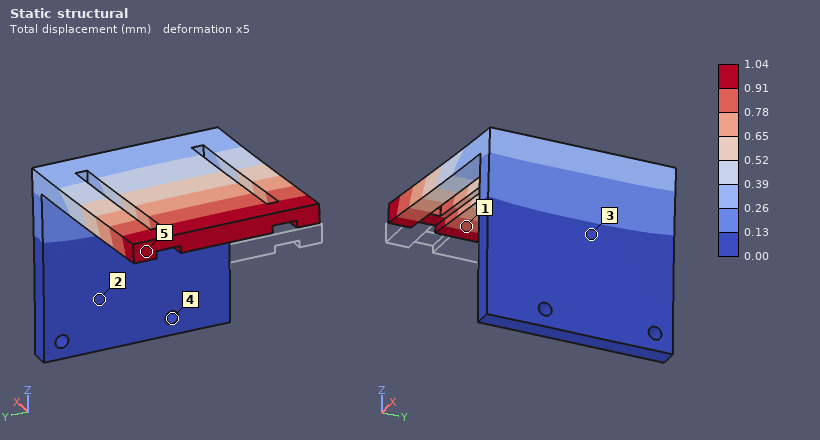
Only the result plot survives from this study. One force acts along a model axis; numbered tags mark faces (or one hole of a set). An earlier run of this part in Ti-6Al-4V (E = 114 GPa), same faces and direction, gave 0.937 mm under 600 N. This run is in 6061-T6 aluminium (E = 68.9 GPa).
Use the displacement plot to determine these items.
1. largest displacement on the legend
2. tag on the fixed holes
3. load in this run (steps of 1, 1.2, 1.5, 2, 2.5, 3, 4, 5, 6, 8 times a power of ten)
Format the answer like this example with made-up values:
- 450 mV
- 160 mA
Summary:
- 1.04 mm
- 4
- 400 N
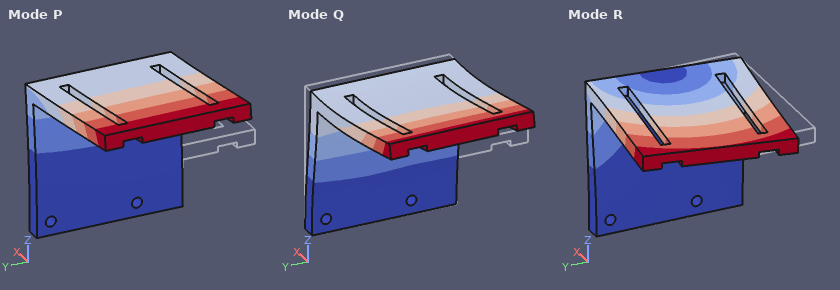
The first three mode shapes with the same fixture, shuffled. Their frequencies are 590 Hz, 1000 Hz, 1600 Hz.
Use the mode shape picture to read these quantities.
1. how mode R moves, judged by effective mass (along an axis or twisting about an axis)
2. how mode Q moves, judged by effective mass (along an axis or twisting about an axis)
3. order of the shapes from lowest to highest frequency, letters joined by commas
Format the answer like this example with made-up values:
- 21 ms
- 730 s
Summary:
- along Y
- along X
- P, R, Q
